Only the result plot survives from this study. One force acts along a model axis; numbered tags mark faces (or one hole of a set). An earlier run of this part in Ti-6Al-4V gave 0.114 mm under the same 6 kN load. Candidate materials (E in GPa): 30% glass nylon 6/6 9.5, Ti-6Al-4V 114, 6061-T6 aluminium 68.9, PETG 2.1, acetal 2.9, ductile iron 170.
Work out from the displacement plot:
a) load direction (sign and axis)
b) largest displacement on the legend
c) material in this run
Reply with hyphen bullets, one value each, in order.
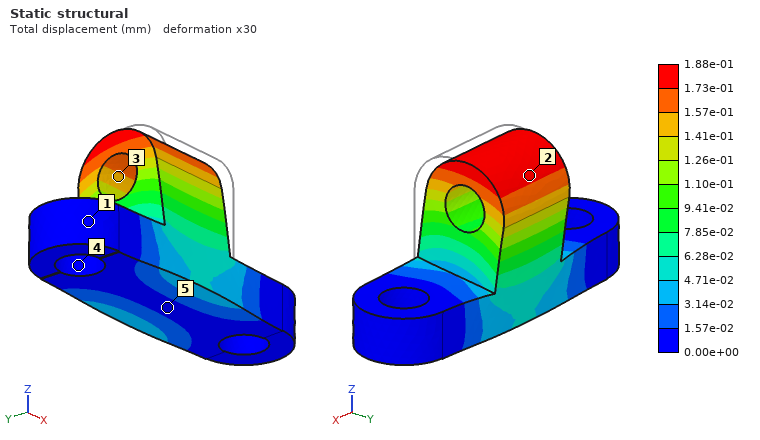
- +Y
- 1.88e-01 mm
- 6061-T6 aluminium
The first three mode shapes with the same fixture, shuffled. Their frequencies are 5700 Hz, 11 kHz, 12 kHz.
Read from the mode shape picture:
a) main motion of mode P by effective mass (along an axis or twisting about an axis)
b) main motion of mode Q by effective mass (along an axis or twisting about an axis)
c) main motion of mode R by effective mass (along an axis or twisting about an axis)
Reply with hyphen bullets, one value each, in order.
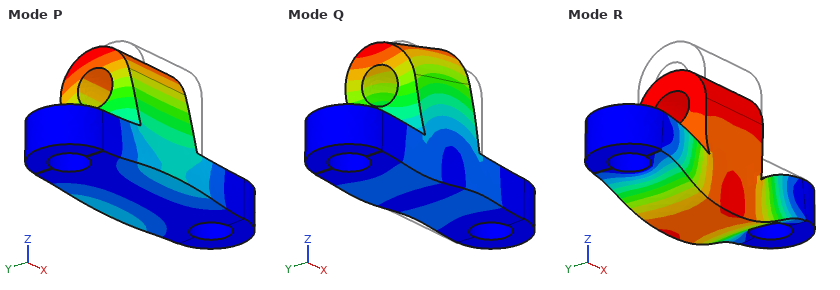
- along Y
- along X
- along Z
